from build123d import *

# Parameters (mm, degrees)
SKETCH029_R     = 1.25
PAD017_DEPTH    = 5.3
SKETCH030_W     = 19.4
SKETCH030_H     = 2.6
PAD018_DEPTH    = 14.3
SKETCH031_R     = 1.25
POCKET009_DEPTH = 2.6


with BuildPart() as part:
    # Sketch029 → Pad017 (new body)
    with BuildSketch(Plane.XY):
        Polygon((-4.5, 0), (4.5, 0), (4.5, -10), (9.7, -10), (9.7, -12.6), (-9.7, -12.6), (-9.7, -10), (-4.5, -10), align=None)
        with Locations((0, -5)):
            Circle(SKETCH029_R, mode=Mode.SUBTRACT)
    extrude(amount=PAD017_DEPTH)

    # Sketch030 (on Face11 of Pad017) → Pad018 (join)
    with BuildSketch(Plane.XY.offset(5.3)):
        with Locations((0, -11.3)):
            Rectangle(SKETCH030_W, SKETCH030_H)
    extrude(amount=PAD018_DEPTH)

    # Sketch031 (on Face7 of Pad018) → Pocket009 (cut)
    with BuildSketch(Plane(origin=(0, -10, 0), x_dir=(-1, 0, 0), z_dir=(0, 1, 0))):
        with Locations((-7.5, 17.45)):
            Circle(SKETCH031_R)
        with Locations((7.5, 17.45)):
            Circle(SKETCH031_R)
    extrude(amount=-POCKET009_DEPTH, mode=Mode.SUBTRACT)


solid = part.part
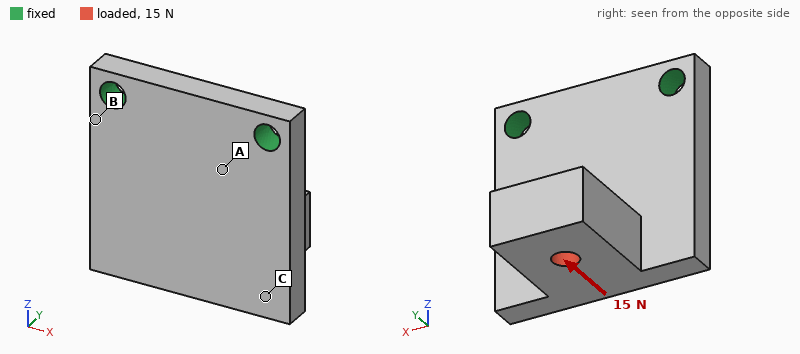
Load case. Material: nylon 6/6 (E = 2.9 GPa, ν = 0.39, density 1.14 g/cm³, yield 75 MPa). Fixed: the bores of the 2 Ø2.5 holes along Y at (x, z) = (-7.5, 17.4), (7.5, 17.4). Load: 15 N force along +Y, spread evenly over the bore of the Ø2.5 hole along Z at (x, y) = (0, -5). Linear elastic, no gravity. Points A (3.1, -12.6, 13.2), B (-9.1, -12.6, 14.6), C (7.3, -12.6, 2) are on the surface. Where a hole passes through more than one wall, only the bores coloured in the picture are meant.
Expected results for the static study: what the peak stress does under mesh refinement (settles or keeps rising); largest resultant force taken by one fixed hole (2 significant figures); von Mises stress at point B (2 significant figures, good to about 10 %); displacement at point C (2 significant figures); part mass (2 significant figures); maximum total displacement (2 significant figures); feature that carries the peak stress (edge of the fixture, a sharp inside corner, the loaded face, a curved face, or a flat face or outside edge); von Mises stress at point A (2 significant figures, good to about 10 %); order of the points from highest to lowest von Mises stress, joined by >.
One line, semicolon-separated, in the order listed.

keeps rising; 7.5 N; 10 MPa; 0.23 mm; 1.6 g; 0.36 mm; edge of the fixture; 5.6 MPa; B > A > C
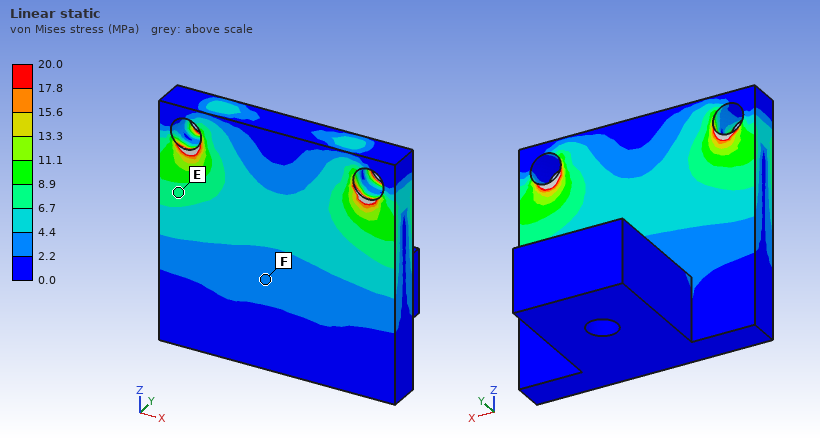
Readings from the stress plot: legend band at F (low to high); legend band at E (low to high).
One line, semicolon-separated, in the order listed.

2.2 to 4.4 MPa; 6.7 to 8.9 MPa
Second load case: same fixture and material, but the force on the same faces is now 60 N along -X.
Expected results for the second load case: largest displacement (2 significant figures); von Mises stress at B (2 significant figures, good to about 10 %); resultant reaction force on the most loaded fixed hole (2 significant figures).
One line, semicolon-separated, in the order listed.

0.34 mm; 16 MPa; 68 N
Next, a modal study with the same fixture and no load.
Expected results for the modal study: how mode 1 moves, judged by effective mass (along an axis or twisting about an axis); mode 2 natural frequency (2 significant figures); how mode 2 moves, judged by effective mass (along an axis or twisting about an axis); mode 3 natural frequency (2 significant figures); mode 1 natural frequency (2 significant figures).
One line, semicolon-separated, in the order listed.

along Y; 3000 Hz; along X; 4700 Hz; 1200 Hz
